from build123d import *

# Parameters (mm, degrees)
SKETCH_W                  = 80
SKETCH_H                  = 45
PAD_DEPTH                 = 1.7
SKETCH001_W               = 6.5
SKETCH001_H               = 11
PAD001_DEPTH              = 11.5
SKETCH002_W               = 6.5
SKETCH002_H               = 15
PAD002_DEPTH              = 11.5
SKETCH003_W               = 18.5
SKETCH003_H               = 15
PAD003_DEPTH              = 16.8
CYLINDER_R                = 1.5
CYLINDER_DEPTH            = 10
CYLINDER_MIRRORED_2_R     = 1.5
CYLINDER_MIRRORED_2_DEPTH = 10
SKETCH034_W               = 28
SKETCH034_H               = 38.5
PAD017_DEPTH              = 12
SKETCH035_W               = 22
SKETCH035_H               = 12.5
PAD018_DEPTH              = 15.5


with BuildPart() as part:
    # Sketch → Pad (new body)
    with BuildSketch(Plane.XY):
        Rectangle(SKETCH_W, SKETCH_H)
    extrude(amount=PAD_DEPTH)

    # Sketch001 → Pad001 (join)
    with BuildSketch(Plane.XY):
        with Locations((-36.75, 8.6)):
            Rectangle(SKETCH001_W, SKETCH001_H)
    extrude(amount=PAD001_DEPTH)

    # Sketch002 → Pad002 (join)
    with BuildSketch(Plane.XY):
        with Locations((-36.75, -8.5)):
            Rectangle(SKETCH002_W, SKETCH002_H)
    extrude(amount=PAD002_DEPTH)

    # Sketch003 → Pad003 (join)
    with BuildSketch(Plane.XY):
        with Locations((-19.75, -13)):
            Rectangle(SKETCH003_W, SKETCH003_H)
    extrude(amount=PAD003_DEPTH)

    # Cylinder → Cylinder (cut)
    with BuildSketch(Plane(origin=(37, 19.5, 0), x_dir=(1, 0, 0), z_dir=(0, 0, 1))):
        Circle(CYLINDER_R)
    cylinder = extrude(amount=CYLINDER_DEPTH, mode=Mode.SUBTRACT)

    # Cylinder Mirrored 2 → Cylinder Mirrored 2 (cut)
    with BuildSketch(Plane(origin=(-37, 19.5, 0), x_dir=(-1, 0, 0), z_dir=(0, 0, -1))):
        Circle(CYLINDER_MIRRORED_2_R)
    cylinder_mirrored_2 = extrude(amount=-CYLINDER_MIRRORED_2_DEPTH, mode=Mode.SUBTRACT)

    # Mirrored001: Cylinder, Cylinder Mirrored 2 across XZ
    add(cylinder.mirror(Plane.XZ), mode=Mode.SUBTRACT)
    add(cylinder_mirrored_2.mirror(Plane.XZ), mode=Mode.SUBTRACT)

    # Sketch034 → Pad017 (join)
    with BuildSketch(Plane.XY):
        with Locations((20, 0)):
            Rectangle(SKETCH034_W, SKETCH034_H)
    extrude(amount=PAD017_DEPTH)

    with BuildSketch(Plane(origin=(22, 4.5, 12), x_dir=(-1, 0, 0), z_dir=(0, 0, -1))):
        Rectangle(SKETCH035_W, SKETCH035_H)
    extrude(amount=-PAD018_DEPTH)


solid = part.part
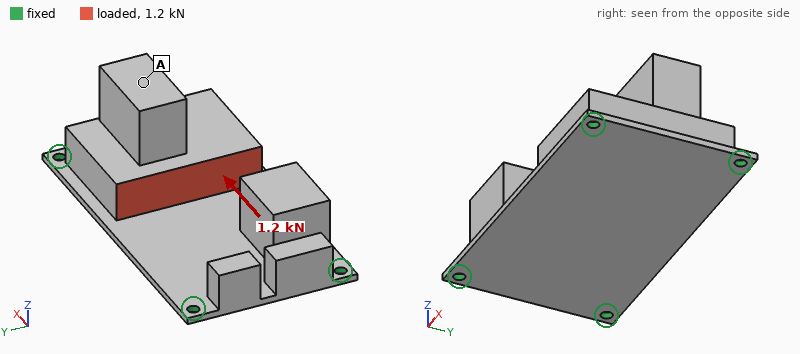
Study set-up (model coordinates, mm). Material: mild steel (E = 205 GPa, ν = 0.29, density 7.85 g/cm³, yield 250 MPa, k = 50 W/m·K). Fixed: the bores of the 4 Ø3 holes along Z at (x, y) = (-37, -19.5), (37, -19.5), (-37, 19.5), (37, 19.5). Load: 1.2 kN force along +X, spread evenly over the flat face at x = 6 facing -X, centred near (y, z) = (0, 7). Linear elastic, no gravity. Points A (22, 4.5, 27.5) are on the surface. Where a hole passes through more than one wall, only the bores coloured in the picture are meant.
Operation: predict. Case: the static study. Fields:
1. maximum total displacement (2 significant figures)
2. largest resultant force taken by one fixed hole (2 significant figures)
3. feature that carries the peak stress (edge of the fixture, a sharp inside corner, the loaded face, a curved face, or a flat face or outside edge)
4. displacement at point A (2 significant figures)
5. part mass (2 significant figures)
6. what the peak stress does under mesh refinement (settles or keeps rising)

0.12 mm
440 N
edge of the fixture
0.10 mm
210 g
keeps rising
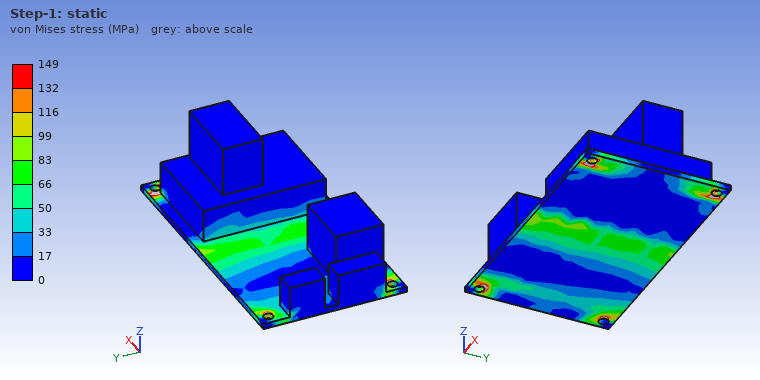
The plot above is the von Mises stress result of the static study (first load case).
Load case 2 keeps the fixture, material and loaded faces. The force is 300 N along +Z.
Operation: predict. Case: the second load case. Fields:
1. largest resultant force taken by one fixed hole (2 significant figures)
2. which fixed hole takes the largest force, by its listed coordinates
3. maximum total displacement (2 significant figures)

100 N
(37, 19.5)
0.15 mm
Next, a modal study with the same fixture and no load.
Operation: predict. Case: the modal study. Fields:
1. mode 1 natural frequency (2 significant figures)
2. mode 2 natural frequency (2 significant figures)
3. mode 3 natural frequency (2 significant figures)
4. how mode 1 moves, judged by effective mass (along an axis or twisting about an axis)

810 Hz
2700 Hz
3400 Hz
along Z
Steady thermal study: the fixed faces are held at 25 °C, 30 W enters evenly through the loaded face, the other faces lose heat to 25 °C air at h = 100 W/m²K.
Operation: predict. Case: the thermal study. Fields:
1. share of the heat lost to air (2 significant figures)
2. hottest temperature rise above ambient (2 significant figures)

71 %
45 K
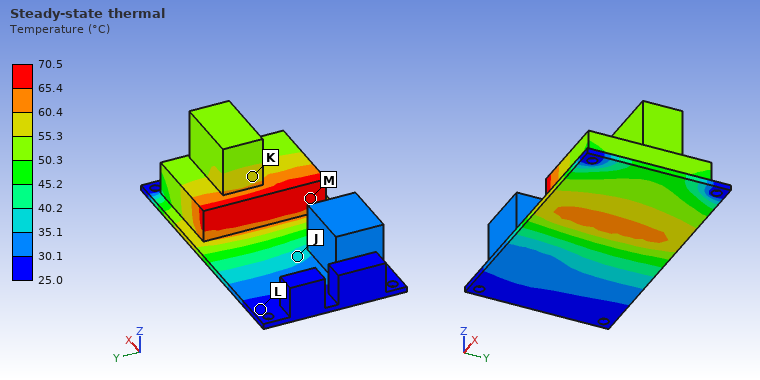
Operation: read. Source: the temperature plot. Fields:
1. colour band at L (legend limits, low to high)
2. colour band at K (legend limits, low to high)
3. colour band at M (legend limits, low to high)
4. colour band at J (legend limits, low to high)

25.0 to 30.1 °C
55.3 to 60.4 °C
65.4 to 70.5 °C
35.1 to 40.2 °C
